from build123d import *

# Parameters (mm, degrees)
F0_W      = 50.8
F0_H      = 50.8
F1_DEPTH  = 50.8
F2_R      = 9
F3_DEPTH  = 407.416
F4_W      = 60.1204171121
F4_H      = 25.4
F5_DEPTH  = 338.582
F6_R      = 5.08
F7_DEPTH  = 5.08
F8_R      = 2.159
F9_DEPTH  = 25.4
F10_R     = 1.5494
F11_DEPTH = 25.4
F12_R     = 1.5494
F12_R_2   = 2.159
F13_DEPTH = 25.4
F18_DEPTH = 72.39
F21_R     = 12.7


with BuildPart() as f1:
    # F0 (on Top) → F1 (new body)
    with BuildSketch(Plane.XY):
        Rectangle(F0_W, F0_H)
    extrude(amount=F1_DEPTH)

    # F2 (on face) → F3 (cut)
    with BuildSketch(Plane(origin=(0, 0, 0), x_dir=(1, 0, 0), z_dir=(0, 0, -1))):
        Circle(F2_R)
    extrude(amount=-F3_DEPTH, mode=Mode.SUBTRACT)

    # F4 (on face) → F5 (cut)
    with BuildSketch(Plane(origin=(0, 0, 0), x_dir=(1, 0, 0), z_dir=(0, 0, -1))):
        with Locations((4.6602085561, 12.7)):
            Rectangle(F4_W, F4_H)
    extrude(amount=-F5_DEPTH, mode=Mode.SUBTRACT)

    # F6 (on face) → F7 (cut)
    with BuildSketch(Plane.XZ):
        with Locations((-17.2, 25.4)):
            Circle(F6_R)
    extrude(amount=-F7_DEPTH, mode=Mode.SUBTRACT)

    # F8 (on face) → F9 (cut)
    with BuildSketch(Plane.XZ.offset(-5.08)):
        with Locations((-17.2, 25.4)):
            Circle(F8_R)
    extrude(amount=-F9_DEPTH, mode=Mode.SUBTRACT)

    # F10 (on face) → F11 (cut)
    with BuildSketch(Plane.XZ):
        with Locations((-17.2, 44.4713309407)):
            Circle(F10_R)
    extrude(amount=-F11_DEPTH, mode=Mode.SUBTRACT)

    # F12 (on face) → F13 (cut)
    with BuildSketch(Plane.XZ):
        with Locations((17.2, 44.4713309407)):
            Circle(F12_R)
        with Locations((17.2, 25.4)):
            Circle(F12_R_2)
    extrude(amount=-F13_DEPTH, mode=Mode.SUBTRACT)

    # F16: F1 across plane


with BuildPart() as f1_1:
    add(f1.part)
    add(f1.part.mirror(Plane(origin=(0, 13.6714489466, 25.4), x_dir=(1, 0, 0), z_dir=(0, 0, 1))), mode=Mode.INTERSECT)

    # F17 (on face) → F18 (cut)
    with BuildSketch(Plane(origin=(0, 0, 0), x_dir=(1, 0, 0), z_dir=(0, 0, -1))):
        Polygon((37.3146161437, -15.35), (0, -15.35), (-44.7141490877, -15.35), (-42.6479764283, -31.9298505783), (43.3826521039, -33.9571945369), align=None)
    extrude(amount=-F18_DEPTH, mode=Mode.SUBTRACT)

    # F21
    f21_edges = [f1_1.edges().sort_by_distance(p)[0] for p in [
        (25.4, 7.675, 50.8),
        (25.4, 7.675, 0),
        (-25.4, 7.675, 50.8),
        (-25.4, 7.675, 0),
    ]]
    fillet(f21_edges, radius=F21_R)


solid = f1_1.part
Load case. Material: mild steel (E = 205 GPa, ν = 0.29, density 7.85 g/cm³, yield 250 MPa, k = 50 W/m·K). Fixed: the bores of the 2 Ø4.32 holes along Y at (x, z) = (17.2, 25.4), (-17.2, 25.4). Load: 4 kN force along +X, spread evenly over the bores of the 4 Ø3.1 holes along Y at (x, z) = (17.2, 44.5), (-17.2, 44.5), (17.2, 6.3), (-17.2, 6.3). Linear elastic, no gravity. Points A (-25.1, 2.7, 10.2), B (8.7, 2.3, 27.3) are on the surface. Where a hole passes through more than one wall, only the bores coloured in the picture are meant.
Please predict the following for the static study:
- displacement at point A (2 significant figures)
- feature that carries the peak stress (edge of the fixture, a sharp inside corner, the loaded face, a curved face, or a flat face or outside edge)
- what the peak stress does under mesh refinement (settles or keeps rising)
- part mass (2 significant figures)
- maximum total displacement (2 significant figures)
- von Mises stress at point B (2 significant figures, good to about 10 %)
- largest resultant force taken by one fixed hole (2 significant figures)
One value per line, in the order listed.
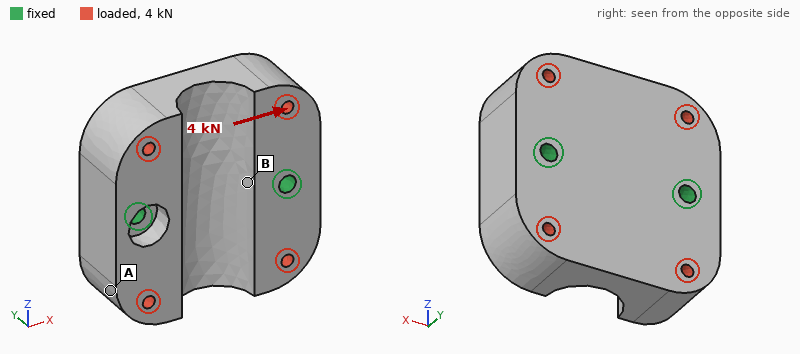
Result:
1.5 µm
edge of the fixture
keeps rising
230 g
2.1 µm
11 MPa
2.0 kN
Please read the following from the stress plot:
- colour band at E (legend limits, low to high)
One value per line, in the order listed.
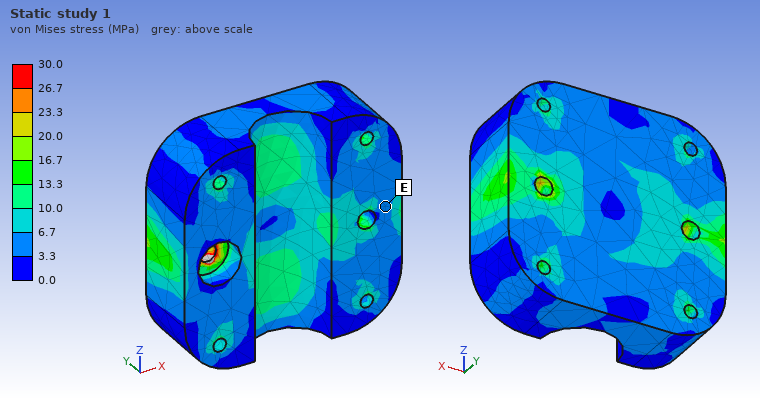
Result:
3.3 to 6.7 MPa
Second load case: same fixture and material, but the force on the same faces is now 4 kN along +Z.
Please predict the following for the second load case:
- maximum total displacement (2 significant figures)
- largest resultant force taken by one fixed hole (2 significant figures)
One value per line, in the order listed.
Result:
1.5 µm
2.0 kN
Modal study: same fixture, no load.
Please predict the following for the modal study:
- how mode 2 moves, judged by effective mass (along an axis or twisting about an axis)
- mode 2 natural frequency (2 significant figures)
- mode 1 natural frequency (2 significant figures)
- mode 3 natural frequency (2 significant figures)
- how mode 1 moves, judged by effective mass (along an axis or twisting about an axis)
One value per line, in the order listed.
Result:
along Y
15 kHz
11 kHz
17 kHz
twisting about X
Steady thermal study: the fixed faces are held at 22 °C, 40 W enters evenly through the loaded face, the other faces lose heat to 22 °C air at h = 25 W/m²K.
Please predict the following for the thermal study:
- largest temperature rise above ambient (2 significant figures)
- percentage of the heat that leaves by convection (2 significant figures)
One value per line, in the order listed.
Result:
19 K
5.3 %
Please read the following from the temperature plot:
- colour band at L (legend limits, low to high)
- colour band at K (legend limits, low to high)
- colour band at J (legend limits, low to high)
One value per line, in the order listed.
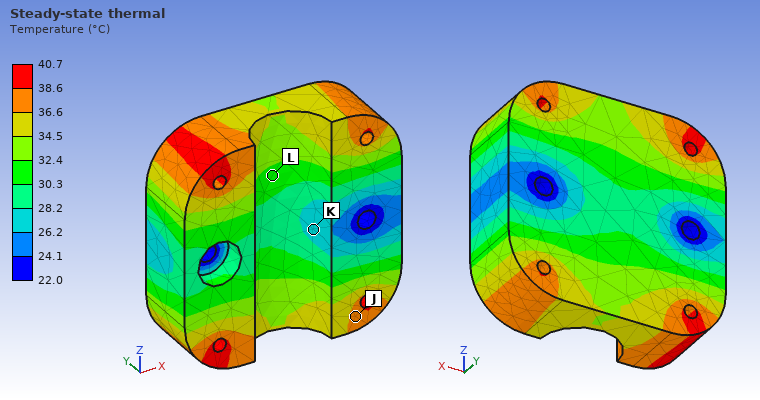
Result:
30.3 to 32.4 °C
26.2 to 28.2 °C
36.6 to 38.6 °C
